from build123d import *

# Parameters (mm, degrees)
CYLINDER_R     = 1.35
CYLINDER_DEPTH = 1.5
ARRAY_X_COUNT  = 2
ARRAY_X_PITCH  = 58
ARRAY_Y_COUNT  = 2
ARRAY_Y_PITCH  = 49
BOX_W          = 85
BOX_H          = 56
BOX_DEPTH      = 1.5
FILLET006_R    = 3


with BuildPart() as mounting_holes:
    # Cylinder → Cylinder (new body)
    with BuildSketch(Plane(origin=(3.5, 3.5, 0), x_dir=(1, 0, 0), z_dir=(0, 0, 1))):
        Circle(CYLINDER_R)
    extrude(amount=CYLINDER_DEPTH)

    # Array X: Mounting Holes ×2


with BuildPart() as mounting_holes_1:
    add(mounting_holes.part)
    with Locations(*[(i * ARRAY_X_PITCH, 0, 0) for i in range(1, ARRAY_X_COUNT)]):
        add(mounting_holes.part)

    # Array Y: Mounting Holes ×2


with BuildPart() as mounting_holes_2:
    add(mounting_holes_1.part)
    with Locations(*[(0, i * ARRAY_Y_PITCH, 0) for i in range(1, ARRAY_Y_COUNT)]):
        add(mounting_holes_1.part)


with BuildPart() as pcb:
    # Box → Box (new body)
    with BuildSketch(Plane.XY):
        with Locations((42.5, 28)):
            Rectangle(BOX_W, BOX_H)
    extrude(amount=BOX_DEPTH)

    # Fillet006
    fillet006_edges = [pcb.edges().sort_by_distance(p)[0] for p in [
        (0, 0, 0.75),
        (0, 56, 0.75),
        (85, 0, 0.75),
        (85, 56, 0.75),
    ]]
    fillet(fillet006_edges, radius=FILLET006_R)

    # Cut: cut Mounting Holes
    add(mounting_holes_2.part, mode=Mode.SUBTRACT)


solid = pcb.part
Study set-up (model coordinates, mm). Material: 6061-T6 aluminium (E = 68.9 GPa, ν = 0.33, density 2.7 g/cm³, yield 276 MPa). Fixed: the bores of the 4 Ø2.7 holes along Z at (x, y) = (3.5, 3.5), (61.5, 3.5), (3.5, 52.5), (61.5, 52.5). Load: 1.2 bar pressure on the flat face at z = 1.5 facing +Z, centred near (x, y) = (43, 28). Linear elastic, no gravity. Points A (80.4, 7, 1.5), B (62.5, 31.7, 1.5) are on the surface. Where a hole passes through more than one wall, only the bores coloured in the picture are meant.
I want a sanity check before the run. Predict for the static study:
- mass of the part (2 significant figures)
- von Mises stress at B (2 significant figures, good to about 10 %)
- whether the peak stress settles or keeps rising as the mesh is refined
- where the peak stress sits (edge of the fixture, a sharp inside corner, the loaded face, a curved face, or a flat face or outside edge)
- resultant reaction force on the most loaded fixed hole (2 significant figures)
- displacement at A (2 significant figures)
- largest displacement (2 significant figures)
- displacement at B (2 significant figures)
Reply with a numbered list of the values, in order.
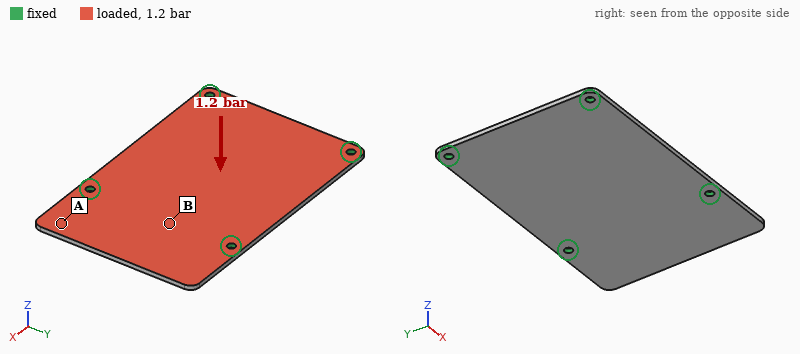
1. 19 g
2. 64 MPa
3. keeps rising
4. edge of the fixture
5. 180 N
6. 0.20 mm
7. 0.38 mm
8. 0.18 mm
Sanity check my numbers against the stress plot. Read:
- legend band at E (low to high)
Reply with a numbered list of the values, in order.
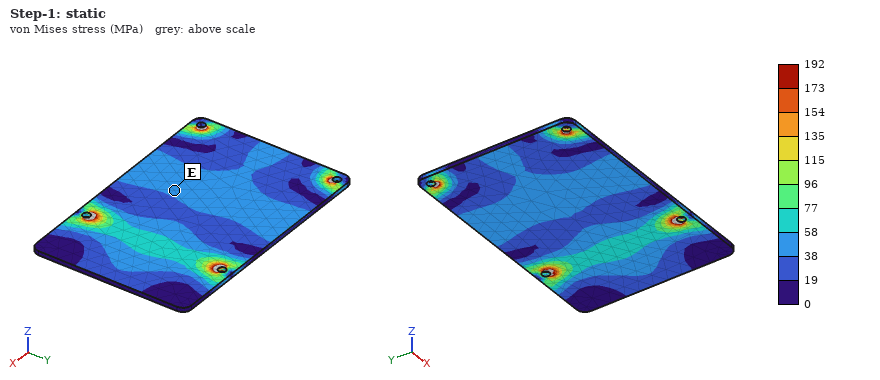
1. 38 to 58 MPa
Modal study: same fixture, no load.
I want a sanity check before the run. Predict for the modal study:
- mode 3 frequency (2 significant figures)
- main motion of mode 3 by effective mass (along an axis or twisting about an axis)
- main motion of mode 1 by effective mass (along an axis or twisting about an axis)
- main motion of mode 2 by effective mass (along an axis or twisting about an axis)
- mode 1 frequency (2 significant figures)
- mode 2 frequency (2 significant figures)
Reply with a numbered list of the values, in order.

1. 2800 Hz
2. twisting about X
3. twisting about Y
4. along Z
5. 1600 Hz
6. 1800 Hz
